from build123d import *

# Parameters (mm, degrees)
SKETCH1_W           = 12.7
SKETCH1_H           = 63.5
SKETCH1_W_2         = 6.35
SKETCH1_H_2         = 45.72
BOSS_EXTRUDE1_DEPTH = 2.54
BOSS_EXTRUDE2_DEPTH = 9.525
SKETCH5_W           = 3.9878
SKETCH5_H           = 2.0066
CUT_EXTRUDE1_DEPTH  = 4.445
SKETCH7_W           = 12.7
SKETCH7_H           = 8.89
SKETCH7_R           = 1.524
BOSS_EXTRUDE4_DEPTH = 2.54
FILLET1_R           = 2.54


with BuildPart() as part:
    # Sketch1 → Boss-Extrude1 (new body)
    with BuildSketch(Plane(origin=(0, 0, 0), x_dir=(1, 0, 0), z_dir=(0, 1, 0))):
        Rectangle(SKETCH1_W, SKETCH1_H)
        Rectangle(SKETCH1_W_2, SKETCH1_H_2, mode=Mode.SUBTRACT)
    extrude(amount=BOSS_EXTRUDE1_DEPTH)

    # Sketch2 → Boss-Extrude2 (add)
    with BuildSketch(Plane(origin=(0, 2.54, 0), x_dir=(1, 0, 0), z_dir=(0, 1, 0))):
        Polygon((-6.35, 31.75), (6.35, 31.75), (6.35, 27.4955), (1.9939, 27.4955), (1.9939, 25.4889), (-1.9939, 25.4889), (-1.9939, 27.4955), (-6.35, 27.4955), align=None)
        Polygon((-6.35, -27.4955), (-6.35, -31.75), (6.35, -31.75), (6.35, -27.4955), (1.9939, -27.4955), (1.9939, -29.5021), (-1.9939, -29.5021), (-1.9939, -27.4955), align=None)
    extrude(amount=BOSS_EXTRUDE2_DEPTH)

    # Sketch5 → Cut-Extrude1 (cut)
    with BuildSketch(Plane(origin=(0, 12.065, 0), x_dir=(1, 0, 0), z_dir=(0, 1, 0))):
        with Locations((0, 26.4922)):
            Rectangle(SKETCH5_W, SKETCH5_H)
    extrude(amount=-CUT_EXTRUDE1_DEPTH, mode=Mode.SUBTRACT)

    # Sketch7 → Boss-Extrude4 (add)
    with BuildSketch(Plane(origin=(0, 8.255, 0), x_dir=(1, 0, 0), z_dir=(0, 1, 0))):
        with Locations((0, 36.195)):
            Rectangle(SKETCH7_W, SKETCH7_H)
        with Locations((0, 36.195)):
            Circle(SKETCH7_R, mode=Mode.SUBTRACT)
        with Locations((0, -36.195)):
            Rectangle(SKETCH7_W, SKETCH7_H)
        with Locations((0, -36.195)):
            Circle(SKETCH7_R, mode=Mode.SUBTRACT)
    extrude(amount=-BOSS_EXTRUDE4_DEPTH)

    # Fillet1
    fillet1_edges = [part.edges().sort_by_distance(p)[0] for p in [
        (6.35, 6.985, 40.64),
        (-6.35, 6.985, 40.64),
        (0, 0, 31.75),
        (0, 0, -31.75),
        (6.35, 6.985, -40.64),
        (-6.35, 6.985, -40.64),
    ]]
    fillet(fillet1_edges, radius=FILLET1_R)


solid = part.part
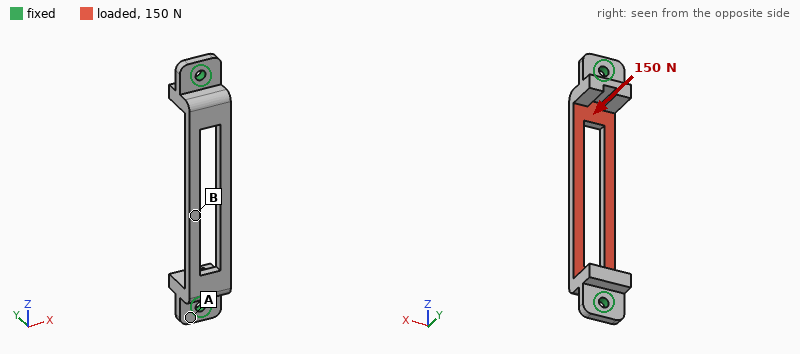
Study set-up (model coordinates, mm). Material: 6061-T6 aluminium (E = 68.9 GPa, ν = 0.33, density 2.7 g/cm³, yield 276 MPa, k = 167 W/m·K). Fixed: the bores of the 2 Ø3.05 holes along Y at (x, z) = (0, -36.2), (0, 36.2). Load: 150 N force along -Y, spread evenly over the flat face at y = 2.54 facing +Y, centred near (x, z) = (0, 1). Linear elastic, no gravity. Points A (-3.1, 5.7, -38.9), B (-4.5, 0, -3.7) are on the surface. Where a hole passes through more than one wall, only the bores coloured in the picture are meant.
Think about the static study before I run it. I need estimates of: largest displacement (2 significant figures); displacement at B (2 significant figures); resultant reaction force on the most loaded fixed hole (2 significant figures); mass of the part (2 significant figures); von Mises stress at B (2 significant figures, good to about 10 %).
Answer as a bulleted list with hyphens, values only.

- 0.10 mm
- 0.099 mm
- 170 N
- 7.5 g
- 50 MPa
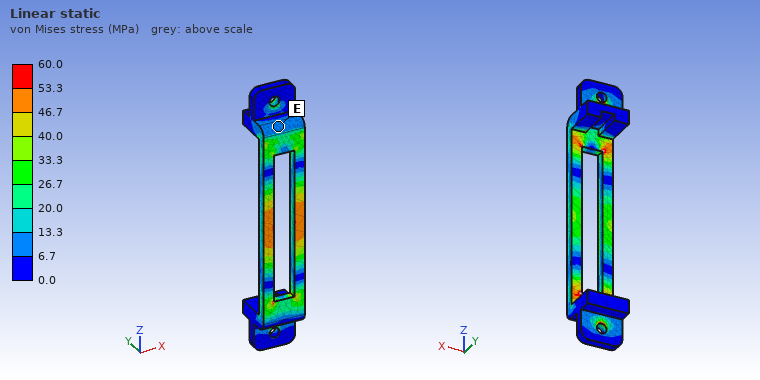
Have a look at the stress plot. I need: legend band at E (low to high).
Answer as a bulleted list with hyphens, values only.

- 6.7 to 13.3 MPa
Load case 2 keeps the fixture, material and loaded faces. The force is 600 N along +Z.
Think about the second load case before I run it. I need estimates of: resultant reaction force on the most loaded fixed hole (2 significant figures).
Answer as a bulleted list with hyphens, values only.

- 300 N
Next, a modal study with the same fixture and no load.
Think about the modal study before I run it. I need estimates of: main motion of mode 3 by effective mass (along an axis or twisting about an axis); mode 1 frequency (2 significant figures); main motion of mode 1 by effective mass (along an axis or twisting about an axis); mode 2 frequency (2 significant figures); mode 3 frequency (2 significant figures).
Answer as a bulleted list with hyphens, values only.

- along X
- 4200 Hz
- along Y
- 4600 Hz
- 5700 Hz
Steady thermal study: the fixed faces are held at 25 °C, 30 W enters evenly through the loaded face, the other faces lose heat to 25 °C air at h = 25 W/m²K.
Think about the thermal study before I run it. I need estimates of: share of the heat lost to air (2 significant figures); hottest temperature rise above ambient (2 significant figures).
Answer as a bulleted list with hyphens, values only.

- 6.3 %
- 81 K
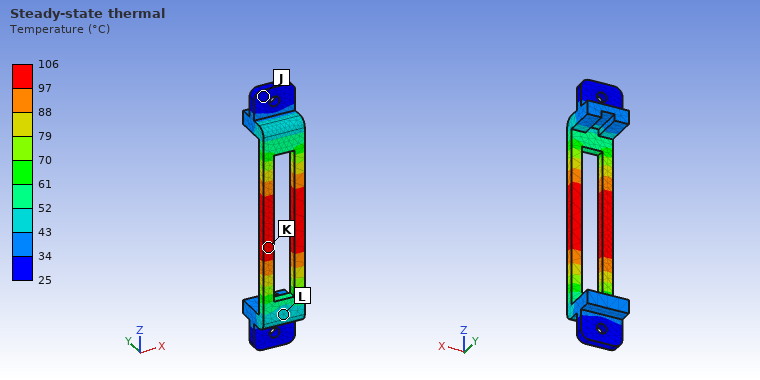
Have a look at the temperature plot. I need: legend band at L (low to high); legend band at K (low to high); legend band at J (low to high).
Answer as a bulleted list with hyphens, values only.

- 43 to 52 °C
- 97 to 106 °C
- 25 to 34 °C
